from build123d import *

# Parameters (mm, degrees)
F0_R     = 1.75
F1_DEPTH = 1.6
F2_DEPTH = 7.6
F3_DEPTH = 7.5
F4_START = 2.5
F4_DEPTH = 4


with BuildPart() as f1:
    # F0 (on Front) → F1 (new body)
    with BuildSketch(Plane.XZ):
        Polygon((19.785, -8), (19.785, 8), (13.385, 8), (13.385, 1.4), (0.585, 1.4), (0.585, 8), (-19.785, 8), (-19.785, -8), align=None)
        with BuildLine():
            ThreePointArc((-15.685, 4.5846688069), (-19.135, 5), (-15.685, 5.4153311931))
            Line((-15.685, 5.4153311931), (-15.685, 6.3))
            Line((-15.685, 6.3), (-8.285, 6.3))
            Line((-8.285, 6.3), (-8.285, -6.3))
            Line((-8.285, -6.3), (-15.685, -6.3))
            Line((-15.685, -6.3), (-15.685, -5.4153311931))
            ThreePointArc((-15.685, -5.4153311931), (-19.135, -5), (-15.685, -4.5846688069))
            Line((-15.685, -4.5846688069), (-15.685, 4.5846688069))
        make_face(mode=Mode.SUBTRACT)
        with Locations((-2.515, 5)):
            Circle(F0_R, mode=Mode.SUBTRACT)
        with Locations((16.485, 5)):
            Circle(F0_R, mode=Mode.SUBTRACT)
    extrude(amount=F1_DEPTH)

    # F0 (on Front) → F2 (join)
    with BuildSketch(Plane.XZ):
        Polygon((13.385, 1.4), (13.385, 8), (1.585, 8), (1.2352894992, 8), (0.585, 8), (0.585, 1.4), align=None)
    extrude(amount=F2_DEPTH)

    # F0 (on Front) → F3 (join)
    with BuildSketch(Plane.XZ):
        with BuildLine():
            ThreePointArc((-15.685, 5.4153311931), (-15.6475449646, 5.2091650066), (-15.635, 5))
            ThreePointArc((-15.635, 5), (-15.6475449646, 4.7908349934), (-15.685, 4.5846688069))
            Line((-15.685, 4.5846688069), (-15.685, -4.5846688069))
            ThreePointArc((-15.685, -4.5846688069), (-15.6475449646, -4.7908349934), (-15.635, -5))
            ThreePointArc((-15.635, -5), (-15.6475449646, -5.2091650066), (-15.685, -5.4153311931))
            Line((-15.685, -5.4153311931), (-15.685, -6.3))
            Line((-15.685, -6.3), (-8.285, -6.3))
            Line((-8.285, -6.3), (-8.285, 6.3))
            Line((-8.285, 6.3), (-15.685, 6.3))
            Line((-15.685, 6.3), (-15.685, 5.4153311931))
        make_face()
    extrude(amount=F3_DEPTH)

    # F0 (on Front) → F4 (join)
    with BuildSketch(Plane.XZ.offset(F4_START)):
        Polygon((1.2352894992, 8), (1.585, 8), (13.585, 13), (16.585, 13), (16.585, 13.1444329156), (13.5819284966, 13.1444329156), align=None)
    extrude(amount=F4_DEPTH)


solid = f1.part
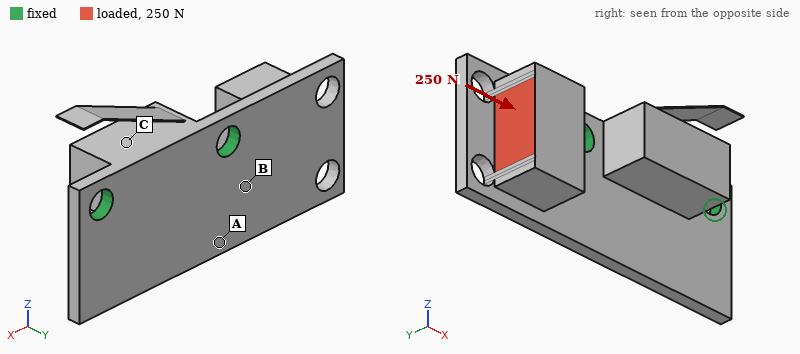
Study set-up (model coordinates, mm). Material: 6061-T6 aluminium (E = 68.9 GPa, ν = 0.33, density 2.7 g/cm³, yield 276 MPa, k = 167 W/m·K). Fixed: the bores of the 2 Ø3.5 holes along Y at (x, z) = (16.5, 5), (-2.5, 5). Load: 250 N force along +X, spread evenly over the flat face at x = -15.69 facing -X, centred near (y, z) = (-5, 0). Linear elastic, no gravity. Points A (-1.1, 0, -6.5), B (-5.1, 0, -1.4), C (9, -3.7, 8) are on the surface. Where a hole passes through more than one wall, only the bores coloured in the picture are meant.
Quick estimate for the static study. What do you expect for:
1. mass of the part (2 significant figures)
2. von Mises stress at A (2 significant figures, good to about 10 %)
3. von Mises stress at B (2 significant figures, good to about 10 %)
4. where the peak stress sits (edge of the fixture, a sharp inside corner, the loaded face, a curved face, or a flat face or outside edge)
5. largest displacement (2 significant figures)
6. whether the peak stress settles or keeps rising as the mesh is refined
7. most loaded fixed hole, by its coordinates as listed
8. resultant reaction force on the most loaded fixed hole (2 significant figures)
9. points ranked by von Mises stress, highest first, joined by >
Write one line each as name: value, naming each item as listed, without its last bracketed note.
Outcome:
mass of the part: 5.4 g
von Mises stress at A: 52 MPa
von Mises stress at B: 91 MPa
where the peak stress sits: edge of the fixture
largest displacement: 0.25 mm
whether the peak stress settles or keeps rising as the mesh is refined: keeps rising
most loaded fixed hole, by its coordinates as listed: (-2.5, 5)
resultant reaction force on the most loaded fixed hole: 180 N
points ranked by von Mises stress, highest first, joined by >: B > A > C
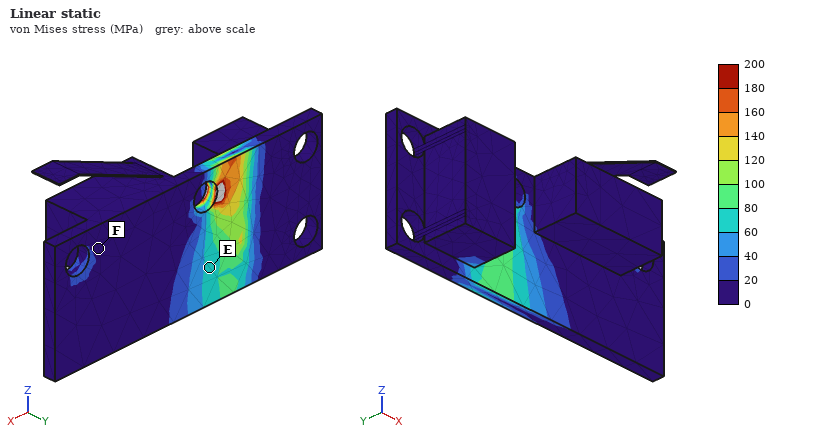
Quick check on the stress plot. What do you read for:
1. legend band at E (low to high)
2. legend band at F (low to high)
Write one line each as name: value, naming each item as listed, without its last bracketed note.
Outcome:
legend band at E: 60 to 80 MPa
legend band at F: 0 to 20 MPa
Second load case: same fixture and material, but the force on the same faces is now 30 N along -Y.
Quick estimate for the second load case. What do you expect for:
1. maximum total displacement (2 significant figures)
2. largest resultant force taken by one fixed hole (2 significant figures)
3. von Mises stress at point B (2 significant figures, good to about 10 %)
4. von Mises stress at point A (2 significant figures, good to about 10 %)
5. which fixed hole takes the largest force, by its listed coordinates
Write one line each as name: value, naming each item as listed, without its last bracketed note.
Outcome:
maximum total displacement: 92 µm
largest resultant force taken by one fixed hole: 35 N
von Mises stress at point B: 32 MPa
von Mises stress at point A: 22 MPa
which fixed hole takes the largest force, by its listed coordinates: (-2.5, 5)
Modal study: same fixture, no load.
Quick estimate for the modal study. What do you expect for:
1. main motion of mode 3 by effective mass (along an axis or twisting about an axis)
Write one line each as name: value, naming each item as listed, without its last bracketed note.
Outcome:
main motion of mode 3 by effective mass: along Y
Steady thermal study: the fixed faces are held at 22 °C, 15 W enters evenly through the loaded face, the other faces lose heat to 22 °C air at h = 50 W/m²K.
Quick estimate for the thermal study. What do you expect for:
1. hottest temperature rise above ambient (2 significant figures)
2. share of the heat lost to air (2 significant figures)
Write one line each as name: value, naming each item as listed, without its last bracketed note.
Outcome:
hottest temperature rise above ambient: 37 K
share of the heat lost to air: 8.5 %
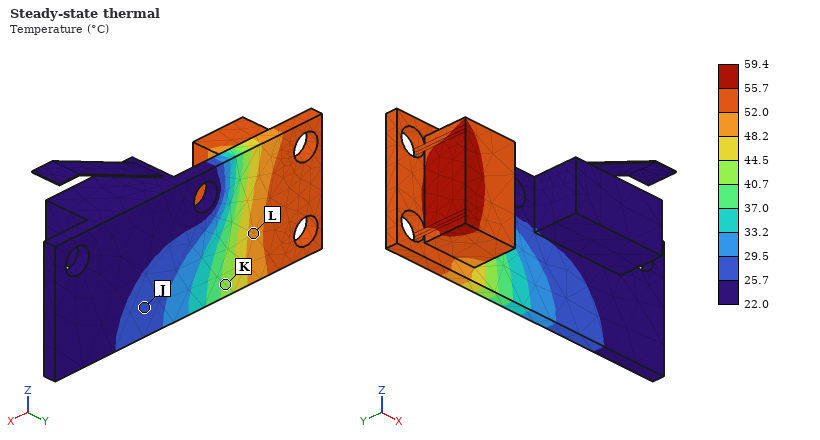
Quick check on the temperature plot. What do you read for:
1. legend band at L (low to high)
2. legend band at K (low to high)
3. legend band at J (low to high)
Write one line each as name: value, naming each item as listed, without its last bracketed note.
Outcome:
legend band at L: 48.2 to 52.0 °C
legend band at K: 40.7 to 44.5 °C
legend band at J: 25.7 to 29.5 °C
